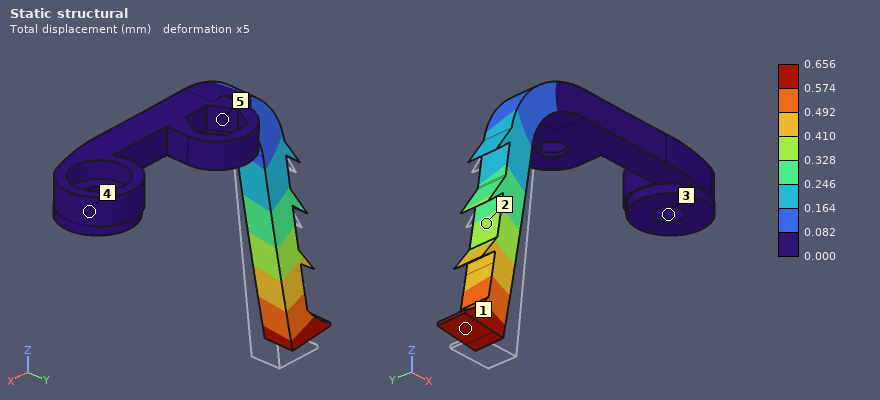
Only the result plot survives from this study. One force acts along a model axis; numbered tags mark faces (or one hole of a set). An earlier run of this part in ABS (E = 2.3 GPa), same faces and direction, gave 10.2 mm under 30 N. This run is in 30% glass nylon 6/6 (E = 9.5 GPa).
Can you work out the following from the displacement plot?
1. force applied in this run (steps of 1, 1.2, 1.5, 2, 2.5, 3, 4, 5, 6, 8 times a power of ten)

8 N
